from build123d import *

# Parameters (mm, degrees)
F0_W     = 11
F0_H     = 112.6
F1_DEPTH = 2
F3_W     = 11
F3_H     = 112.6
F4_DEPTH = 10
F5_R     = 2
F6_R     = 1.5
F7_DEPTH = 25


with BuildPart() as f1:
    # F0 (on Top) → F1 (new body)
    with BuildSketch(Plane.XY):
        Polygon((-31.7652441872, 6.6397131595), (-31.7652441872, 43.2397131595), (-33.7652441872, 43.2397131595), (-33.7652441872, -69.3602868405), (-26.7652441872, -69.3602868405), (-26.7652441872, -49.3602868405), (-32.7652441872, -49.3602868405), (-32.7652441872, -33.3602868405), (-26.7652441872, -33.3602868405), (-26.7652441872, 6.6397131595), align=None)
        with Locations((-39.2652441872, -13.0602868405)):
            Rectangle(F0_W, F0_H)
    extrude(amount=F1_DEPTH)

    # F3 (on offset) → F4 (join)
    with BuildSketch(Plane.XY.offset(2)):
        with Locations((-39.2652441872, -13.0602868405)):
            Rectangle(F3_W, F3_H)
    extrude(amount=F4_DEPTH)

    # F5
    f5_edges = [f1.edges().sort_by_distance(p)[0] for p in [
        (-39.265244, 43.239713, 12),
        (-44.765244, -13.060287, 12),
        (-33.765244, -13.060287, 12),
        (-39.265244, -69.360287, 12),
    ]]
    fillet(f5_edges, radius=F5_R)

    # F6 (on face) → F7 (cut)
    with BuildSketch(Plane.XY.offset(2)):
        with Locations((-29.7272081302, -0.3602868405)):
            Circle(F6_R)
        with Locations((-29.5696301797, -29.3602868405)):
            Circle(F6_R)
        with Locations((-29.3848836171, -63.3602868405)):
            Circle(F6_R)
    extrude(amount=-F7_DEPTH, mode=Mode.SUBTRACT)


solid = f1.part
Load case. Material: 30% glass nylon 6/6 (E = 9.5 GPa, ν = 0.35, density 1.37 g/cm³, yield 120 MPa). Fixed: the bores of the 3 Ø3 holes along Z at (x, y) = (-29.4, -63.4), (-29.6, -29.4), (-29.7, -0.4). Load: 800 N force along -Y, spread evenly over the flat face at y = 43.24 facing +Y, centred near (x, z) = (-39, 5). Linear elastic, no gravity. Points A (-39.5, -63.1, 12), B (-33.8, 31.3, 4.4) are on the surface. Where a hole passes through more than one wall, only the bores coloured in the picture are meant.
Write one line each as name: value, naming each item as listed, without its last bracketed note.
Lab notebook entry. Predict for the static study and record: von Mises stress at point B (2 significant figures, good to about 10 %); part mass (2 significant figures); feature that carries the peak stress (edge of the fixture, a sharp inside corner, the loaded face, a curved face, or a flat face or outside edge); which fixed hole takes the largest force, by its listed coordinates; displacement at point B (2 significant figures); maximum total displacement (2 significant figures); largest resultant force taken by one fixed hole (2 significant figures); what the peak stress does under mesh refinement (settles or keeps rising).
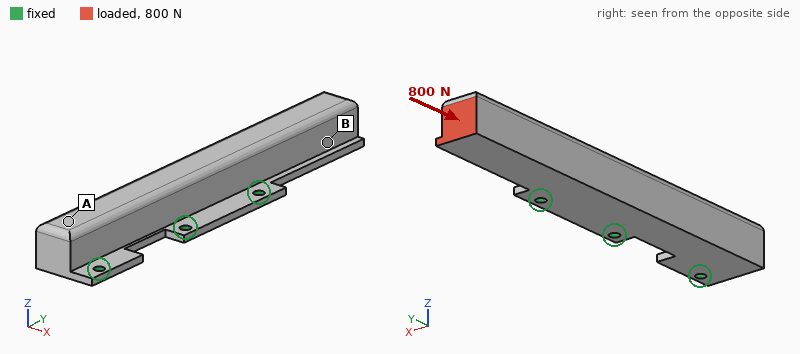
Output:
von Mises stress at point B: 6.6 MPa
part mass: 21 g
feature that carries the peak stress: edge of the fixture
which fixed hole takes the largest force, by its listed coordinates: (-29.7, -0.4)
displacement at point B: 0.069 mm
maximum total displacement: 0.11 mm
largest resultant force taken by one fixed hole: 390 N
what the peak stress does under mesh refinement: keeps rising
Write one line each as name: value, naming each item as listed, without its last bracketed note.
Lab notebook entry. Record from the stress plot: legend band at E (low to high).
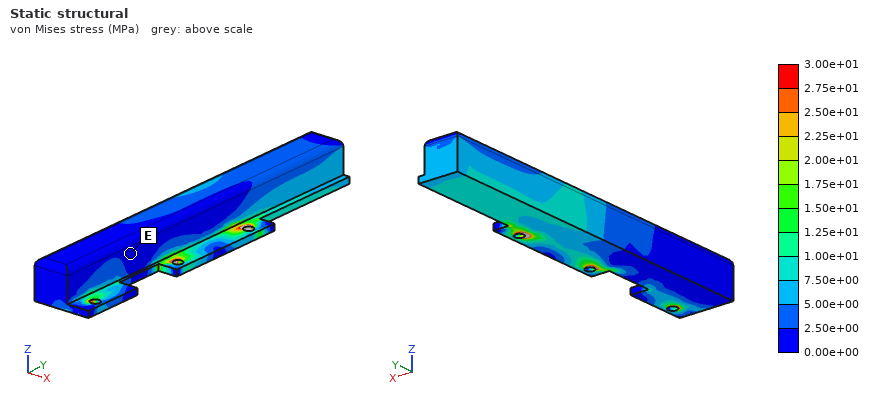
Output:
legend band at E: 0.00e+00 to 2.50e+00 MPa
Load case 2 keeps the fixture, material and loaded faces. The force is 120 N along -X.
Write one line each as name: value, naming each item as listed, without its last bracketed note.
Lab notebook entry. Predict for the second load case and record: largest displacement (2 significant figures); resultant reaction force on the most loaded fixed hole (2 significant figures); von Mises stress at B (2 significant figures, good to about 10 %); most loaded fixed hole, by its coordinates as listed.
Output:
largest displacement: 0.52 mm
resultant reaction force on the most loaded fixed hole: 310 N
von Mises stress at B: 5.2 MPa
most loaded fixed hole, by its coordinates as listed: (-29.7, -0.4)
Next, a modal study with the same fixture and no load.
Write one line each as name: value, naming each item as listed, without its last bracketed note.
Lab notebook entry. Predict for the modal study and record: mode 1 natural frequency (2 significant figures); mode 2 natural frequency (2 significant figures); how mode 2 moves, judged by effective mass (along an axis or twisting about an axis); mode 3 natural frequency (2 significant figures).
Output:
mode 1 natural frequency: 840 Hz
mode 2 natural frequency: 1500 Hz
how mode 2 moves, judged by effective mass: twisting about X
mode 3 natural frequency: 2100 Hz
